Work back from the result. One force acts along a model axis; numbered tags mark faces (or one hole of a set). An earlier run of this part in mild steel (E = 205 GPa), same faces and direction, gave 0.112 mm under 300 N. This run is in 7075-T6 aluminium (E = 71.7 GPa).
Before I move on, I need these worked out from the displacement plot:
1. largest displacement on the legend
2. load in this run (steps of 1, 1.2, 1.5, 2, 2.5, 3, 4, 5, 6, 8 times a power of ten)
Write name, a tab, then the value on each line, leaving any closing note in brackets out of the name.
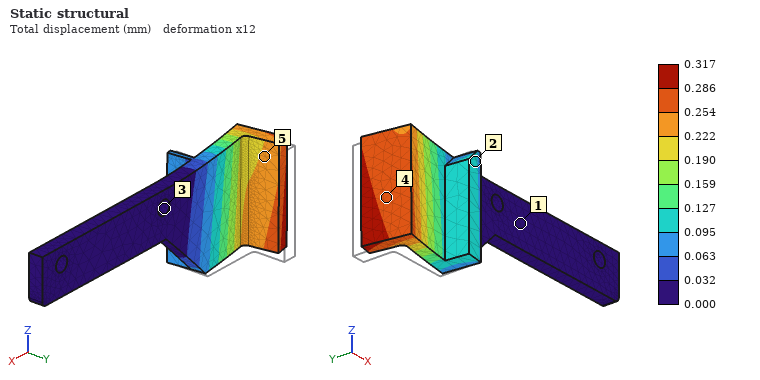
largest displacement on the legend	0.317 mm
load in this run	300 N
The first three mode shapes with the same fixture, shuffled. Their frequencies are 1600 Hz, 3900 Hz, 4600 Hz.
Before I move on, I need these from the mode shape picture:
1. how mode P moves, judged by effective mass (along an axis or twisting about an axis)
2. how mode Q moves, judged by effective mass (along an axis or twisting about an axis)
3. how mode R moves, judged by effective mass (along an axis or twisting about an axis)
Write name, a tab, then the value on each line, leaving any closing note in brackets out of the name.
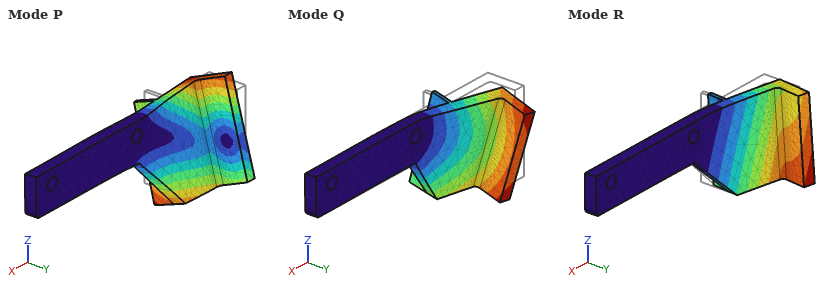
how mode P moves, judged by effective mass	along Z
how mode Q moves, judged by effective mass	along Z
how mode R moves, judged by effective mass	along Y
